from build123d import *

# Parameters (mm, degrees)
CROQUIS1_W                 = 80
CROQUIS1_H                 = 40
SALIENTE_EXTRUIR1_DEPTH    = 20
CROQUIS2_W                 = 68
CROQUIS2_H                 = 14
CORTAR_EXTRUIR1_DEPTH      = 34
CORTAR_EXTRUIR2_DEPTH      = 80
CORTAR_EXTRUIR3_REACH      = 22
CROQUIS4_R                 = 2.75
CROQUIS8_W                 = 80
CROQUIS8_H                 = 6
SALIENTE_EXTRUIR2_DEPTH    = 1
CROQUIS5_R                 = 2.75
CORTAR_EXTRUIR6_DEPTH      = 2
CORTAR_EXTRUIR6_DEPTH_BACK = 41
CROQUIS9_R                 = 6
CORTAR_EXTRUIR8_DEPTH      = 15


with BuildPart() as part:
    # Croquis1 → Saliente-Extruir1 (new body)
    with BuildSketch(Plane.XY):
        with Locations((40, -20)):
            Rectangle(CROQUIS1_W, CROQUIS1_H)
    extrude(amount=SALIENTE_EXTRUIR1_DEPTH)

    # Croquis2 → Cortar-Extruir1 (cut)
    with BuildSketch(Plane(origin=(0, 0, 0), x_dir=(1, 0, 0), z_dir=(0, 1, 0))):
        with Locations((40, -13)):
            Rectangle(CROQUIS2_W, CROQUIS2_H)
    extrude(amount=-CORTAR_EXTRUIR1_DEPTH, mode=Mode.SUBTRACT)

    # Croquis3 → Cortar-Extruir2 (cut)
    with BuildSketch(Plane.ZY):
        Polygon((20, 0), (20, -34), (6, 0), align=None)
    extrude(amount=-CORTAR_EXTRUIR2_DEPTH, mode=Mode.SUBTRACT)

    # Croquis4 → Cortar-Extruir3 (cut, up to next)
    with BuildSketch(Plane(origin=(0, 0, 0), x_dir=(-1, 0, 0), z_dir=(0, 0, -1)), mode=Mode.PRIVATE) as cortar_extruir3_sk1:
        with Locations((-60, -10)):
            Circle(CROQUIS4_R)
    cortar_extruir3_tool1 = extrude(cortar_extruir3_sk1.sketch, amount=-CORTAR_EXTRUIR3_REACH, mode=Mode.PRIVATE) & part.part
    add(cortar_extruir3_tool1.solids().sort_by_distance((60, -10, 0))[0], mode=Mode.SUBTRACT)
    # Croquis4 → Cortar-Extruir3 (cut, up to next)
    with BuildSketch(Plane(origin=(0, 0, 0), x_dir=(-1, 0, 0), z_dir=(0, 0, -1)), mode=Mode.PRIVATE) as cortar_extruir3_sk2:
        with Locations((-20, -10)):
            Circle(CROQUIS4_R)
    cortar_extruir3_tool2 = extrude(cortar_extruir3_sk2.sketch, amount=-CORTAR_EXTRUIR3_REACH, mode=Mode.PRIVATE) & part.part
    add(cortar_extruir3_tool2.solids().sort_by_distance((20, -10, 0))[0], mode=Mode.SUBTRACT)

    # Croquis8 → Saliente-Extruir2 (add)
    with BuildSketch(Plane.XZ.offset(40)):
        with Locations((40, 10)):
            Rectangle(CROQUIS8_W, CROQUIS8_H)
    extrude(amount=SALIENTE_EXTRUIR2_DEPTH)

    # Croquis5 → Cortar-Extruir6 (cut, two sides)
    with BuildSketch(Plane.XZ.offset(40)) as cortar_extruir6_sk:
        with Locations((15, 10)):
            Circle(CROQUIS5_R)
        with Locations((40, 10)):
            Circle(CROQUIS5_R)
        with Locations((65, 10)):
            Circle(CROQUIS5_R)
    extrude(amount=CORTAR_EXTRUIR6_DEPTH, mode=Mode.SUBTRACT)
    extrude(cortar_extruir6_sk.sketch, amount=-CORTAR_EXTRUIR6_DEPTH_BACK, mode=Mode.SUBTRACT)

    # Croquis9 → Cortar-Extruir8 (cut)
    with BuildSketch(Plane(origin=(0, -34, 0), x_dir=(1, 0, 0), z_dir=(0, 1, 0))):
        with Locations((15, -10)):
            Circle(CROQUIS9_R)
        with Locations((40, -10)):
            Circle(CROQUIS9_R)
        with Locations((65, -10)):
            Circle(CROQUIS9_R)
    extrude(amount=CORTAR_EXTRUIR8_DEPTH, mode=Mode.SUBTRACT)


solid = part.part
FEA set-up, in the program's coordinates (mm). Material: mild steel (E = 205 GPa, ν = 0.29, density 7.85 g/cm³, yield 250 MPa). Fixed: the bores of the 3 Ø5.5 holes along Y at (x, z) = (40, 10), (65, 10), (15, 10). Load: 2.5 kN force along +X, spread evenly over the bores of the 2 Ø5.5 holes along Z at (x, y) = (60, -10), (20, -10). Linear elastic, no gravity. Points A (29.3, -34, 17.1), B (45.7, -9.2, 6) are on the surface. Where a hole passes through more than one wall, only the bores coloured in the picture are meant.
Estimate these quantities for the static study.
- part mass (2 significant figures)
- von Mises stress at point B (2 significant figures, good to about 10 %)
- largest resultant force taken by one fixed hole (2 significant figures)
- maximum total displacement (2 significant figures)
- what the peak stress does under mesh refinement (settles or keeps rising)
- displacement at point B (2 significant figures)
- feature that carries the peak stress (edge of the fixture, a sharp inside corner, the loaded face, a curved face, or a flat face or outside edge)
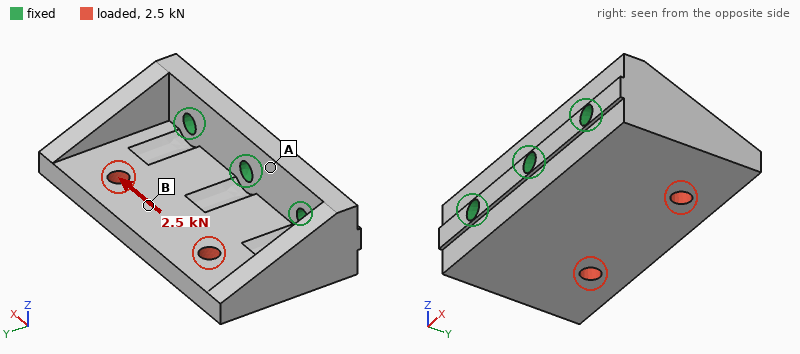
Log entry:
220 g
12 MPa
1.5 kN
11 µm
keeps rising
5.6 µm
edge of the fixture
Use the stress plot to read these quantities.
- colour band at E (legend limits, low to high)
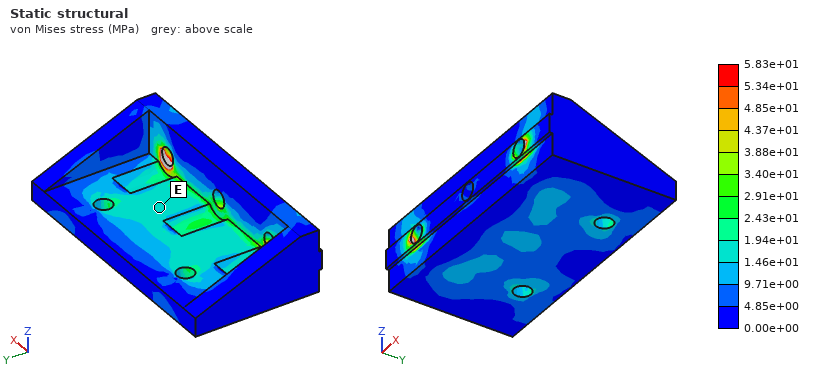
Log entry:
1.46e+01 to 1.94e+01 MPa
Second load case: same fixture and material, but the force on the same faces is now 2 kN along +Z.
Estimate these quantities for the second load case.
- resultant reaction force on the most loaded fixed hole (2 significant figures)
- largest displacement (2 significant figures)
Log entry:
770 N
70 µm
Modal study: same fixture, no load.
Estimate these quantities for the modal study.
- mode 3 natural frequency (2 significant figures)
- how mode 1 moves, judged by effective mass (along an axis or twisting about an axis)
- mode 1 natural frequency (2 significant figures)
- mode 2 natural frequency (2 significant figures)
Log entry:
9000 Hz
along Z
3700 Hz
5200 Hz
